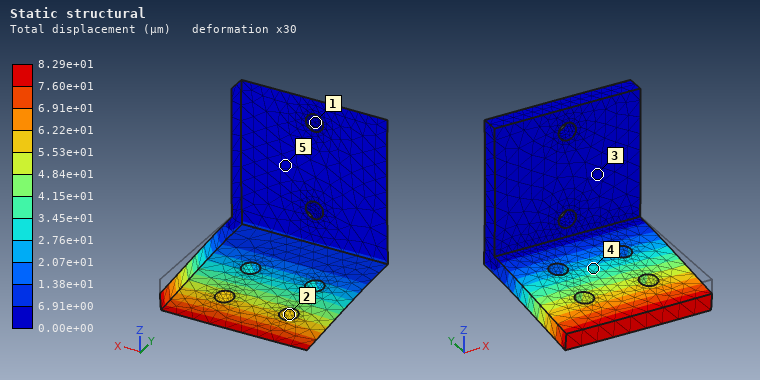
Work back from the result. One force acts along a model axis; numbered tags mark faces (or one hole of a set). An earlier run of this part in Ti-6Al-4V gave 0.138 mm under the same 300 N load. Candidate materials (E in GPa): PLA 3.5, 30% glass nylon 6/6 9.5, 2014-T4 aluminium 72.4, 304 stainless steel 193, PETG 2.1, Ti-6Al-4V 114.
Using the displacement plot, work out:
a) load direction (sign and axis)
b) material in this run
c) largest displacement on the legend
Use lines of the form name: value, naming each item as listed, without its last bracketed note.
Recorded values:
load direction: -Z
material in this run: 304 stainless steel
largest displacement on the legend: 8.29e+01 µm
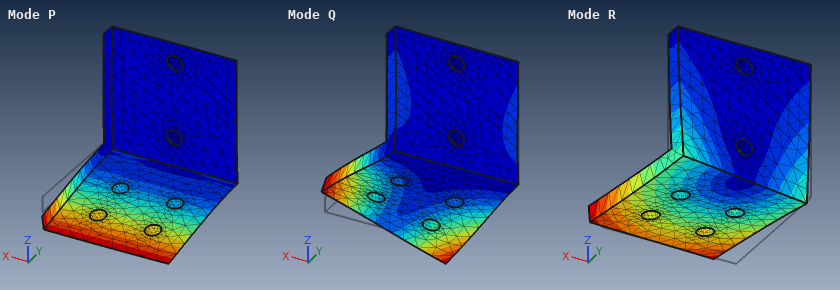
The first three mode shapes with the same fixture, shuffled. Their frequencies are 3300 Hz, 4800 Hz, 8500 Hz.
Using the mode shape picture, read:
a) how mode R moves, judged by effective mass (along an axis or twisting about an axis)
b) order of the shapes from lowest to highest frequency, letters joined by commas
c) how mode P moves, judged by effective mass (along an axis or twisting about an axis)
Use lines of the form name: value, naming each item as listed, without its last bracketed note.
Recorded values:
how mode R moves, judged by effective mass: along X
order of the shapes from lowest to highest frequency, letters joined by commas: P, R, Q
how mode P moves, judged by effective mass: along Z
